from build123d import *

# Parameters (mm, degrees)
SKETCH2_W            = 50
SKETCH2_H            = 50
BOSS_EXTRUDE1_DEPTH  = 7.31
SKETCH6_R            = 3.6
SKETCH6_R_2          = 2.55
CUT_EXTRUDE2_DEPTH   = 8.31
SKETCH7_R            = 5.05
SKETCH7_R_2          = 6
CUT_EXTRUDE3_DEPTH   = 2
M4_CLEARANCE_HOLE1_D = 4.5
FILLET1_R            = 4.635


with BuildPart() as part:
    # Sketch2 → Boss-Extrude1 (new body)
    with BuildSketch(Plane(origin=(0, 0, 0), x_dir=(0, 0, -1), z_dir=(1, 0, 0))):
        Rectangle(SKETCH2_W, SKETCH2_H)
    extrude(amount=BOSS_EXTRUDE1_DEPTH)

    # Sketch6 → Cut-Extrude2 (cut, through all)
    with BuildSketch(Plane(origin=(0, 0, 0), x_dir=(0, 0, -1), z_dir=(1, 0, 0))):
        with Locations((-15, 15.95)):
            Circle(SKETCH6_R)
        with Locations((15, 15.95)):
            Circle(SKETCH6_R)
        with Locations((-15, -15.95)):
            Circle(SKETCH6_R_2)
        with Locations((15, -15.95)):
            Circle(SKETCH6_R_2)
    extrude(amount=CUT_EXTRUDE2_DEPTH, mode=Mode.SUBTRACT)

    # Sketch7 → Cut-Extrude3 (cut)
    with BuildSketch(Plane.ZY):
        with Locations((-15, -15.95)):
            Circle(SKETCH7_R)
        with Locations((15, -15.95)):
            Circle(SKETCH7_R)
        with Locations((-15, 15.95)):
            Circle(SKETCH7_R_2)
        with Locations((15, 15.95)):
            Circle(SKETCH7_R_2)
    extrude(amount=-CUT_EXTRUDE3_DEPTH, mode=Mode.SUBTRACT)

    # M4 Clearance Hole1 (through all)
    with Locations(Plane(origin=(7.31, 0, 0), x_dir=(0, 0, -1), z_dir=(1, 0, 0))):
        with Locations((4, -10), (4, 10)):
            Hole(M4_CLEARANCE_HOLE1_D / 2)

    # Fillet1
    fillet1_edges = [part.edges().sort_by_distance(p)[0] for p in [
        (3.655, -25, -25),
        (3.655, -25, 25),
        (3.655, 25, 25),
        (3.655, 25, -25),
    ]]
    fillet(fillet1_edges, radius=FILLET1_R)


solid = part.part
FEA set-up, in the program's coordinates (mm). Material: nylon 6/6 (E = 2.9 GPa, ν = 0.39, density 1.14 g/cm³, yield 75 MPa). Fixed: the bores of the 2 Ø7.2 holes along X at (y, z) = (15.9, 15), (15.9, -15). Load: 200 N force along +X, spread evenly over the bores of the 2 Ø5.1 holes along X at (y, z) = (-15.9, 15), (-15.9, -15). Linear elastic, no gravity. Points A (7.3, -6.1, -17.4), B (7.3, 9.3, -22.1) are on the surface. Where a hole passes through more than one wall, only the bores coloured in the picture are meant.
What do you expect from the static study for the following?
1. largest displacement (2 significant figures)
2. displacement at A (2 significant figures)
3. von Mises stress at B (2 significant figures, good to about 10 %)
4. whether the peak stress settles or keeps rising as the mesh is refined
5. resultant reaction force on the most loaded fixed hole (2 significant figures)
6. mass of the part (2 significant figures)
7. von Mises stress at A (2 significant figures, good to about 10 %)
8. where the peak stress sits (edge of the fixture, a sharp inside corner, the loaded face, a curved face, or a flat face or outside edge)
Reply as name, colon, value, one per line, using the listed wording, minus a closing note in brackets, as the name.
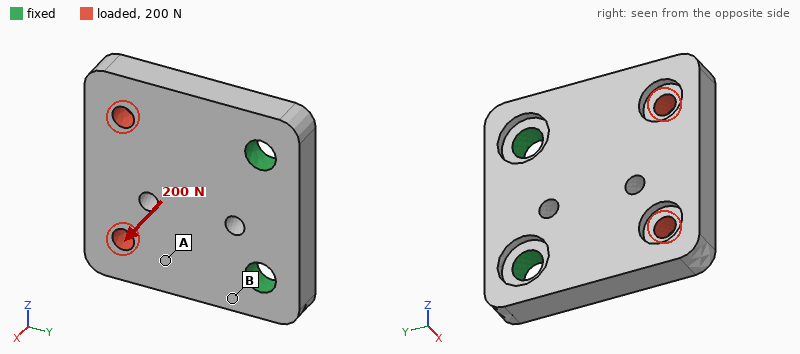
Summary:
largest displacement: 0.82 mm
displacement at A: 0.34 mm
von Mises stress at B: 12 MPa
whether the peak stress settles or keeps rising as the mesh is refined: keeps rising
resultant reaction force on the most loaded fixed hole: 100 N
mass of the part: 19 g
von Mises stress at A: 4.7 MPa
where the peak stress sits: edge of the fixture
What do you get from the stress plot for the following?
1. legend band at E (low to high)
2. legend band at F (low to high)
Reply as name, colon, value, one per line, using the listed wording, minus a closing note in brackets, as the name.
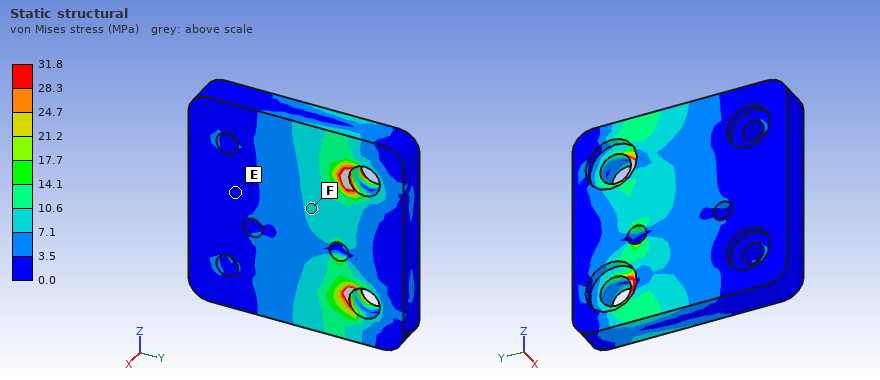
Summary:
legend band at E: 0.0 to 3.5 MPa
legend band at F: 7.1 to 10.6 MPa
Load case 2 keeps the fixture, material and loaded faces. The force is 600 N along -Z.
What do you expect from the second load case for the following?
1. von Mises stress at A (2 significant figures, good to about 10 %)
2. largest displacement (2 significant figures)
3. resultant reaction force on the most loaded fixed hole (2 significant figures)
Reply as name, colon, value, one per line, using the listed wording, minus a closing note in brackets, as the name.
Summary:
von Mises stress at A: 4.0 MPa
largest displacement: 0.16 mm
resultant reaction force on the most loaded fixed hole: 620 N
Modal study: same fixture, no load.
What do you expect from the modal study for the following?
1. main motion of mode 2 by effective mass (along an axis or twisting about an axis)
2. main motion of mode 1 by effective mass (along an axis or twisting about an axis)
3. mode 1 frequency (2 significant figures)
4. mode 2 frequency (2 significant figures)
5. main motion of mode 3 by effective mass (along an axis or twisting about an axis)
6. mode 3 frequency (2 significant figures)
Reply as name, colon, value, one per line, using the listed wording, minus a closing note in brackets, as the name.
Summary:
main motion of mode 2 by effective mass: twisting about Y
main motion of mode 1 by effective mass: along X
mode 1 frequency: 1000 Hz
mode 2 frequency: 2100 Hz
main motion of mode 3 by effective mass: along Z
mode 3 frequency: 4000 Hz
